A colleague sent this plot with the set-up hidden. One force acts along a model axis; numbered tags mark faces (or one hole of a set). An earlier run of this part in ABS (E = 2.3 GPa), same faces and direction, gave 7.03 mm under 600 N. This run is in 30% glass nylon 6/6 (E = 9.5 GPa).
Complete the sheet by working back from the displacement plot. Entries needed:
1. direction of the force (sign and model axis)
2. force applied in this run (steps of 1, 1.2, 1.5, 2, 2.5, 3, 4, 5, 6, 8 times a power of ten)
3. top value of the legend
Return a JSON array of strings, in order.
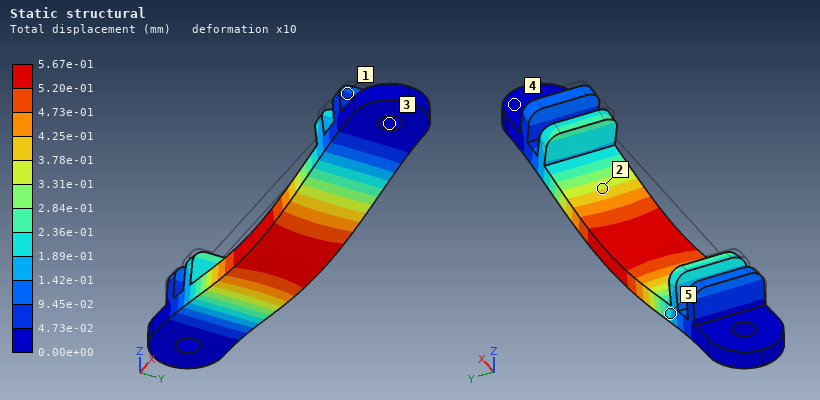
["-Z", "200 N", "5.67e-01 mm"]
